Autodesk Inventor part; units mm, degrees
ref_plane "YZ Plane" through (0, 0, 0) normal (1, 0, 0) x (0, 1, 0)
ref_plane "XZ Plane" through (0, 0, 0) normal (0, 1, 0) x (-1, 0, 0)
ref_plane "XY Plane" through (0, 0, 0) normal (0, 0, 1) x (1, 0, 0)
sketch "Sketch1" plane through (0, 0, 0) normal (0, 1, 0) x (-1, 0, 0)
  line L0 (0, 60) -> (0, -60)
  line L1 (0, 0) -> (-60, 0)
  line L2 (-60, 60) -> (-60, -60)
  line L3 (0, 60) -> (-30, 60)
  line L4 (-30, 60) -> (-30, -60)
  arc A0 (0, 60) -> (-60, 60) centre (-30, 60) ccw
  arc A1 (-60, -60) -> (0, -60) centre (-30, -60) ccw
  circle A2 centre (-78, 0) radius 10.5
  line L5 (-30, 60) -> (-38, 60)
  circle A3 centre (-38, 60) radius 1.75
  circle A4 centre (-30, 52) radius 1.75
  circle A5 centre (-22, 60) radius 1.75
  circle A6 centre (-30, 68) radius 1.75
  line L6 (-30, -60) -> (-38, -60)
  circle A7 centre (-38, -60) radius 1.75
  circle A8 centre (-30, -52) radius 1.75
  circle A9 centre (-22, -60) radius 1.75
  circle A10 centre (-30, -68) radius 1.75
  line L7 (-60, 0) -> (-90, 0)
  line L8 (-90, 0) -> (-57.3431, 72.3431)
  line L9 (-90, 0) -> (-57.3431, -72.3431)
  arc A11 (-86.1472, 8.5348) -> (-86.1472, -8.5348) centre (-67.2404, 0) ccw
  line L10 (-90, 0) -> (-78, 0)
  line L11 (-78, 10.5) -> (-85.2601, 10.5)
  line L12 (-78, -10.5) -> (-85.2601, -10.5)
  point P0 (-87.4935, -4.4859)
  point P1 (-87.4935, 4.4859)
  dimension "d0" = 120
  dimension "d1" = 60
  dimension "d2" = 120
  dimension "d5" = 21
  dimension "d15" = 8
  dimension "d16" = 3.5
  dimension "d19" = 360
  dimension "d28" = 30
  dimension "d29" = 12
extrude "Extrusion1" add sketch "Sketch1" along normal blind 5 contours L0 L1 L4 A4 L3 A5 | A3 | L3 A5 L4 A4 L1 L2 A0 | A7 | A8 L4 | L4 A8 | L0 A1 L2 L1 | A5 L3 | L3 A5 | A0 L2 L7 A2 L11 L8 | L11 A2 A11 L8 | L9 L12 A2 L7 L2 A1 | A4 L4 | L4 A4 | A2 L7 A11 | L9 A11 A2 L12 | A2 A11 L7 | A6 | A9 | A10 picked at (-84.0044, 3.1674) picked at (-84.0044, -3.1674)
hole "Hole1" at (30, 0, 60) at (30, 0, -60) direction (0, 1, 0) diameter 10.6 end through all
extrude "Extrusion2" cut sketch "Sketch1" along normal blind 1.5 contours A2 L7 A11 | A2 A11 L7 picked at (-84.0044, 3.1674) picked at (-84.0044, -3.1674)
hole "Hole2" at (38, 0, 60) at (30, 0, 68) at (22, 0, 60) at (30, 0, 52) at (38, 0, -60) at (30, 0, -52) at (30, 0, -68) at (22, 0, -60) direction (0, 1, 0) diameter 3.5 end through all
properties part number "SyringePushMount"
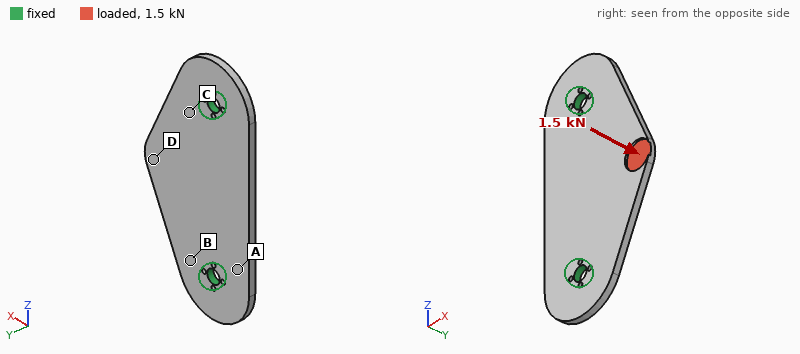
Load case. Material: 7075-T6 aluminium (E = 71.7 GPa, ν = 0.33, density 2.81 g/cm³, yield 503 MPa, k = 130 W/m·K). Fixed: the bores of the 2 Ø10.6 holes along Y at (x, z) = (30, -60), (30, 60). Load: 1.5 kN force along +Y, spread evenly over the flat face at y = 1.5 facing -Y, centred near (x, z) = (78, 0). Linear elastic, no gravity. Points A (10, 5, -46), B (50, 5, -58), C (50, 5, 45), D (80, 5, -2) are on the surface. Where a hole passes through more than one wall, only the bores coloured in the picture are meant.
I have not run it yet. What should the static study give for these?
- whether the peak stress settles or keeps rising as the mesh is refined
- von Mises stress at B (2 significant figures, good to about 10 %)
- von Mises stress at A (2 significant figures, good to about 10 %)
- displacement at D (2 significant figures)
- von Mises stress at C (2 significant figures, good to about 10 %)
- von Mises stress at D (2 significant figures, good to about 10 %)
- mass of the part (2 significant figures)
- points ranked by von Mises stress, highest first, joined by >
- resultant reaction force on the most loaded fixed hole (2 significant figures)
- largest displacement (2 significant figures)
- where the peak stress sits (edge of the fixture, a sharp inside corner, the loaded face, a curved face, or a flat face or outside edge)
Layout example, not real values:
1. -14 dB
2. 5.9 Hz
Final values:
1. keeps rising
2. 120 MPa
3. 45 MPa
4. 1.6 mm
5. 92 MPa
6. 160 MPa
7. 160 g
8. D > B > C > A
9. 760 N
10. 1.9 mm
11. edge of the fixture
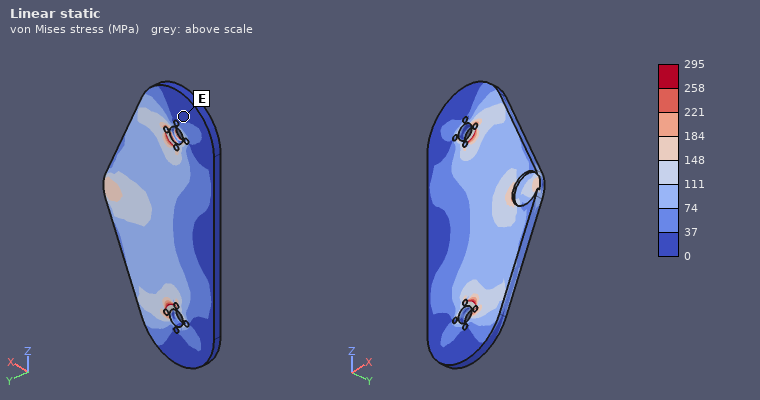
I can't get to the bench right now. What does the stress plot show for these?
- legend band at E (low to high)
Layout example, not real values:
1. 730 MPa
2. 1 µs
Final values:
1. 0 to 37 MPa
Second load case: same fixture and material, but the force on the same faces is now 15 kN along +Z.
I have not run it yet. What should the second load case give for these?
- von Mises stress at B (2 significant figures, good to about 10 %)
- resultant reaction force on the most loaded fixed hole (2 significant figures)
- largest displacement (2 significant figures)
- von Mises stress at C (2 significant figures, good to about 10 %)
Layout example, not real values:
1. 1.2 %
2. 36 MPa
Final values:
1. 52 MPa
2. 9.5 kN
3. 0.18 mm
4. 59 MPa
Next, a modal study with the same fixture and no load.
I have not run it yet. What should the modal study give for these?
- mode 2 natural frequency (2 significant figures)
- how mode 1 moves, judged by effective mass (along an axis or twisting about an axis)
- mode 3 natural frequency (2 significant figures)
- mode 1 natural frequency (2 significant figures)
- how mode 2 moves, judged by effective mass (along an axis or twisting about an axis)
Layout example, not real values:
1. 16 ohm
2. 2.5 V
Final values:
1. 1800 Hz
2. along Y
3. 3100 Hz
4. 1200 Hz
5. along Y
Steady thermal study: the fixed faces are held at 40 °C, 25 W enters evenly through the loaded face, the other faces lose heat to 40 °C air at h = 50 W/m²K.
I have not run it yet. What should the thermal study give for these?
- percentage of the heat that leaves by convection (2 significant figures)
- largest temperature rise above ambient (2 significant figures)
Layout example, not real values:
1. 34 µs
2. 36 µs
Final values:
1. 37 %
2. 35 K
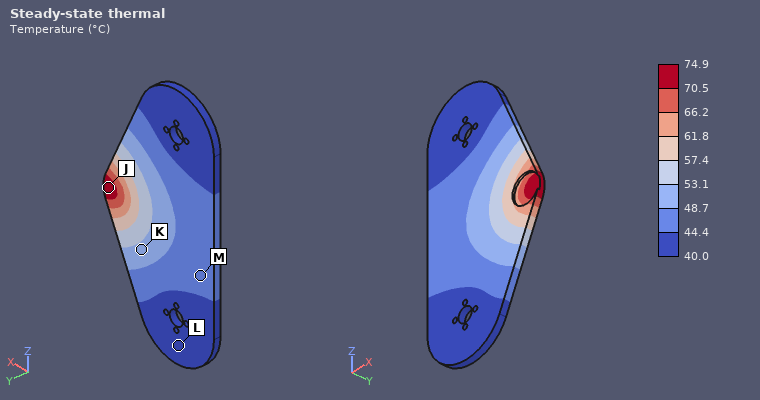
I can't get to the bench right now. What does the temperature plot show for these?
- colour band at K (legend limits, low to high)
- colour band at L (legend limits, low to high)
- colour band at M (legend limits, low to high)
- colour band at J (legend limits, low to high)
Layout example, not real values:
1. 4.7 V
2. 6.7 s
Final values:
1. 48.7 to 53.1 °C
2. 40.0 to 44.4 °C
3. 44.4 to 48.7 °C
4. 70.5 to 74.9 °C
